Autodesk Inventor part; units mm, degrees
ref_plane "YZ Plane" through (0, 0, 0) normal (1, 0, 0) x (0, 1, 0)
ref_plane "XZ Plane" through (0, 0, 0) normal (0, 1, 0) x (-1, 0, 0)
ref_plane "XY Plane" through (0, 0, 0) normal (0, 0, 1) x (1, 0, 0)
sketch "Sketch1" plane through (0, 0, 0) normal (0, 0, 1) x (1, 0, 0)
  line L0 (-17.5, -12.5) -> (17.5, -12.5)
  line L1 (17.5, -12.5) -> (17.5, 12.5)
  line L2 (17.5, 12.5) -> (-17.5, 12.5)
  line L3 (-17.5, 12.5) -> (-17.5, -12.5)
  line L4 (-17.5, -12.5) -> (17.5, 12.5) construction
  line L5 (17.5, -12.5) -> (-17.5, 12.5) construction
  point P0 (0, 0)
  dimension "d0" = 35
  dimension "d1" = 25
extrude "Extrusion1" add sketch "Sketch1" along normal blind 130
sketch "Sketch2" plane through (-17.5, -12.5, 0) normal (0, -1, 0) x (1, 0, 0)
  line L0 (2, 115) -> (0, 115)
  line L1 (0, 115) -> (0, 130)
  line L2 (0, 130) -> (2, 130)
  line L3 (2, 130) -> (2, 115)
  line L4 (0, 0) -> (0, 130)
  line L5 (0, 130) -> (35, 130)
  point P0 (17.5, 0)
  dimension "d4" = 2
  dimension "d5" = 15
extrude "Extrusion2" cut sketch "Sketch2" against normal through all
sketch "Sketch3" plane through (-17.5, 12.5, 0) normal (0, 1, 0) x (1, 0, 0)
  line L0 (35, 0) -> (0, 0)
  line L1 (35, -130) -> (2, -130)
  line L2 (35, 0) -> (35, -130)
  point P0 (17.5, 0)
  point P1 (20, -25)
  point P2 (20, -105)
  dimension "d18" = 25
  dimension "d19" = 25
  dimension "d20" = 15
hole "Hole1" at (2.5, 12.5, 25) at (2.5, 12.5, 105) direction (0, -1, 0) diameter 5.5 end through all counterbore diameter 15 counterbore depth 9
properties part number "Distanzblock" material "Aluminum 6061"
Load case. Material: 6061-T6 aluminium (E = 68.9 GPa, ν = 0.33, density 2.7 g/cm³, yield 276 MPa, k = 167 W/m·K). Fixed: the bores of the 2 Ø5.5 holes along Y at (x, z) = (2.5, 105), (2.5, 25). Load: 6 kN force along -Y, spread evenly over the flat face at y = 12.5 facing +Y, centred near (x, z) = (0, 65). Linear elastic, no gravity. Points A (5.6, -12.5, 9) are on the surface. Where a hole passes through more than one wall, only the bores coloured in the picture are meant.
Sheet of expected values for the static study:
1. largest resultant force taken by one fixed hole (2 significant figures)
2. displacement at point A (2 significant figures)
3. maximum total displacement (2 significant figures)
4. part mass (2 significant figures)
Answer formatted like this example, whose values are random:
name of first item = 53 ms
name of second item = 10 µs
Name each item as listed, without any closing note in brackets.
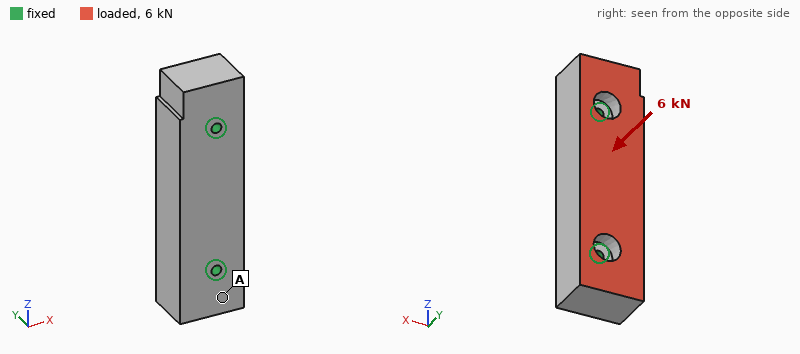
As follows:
largest resultant force taken by one fixed hole = 3.1 kN
displacement at point A = 1.6 µm
maximum total displacement = 8.4 µm
part mass = 290 g
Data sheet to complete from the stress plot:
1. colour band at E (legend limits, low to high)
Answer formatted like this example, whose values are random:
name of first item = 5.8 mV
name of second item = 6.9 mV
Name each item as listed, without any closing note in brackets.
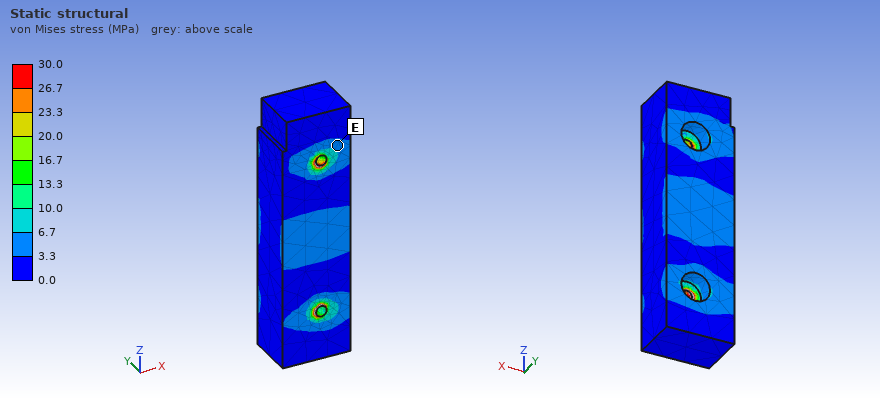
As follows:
colour band at E = 3.3 to 6.7 MPa
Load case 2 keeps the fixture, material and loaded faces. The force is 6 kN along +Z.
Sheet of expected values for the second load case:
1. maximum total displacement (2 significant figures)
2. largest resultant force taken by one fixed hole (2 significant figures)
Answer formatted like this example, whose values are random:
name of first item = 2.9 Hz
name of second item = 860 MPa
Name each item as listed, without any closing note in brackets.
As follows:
maximum total displacement = 7.5 µm
largest resultant force taken by one fixed hole = 3.2 kN
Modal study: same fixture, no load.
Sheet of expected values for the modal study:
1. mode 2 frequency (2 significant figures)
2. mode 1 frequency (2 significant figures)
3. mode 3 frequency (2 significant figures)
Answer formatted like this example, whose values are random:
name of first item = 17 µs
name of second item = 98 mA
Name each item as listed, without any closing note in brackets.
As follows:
mode 2 frequency = 9500 Hz
mode 1 frequency = 8300 Hz
mode 3 frequency = 9900 Hz
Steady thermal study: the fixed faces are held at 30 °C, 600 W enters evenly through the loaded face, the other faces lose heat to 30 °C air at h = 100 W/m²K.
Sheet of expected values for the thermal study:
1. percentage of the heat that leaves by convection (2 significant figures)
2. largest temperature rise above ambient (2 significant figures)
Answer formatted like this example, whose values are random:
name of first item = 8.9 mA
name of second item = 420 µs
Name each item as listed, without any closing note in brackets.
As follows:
percentage of the heat that leaves by convection = 7.1 %
largest temperature rise above ambient = 53 K
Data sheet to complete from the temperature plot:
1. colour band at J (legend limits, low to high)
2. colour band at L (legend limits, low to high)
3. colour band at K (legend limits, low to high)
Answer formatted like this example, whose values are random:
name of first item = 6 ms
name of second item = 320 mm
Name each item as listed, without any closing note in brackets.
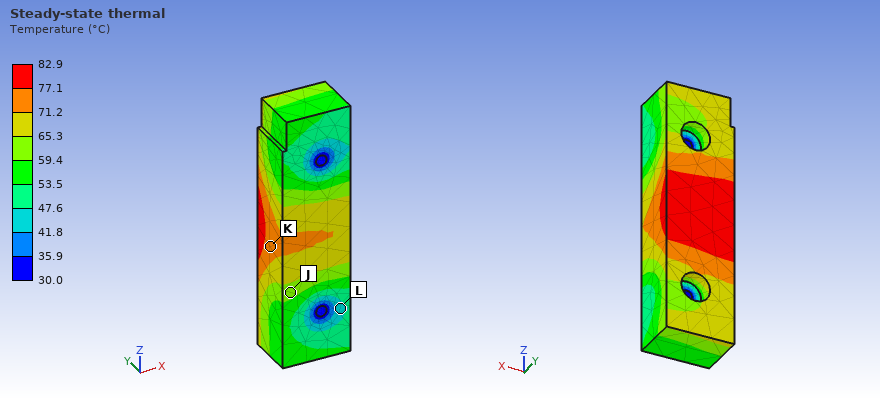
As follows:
colour band at J = 59.4 to 65.3 °C
colour band at L = 41.8 to 47.6 °C
colour band at K = 71.2 to 77.1 °C
